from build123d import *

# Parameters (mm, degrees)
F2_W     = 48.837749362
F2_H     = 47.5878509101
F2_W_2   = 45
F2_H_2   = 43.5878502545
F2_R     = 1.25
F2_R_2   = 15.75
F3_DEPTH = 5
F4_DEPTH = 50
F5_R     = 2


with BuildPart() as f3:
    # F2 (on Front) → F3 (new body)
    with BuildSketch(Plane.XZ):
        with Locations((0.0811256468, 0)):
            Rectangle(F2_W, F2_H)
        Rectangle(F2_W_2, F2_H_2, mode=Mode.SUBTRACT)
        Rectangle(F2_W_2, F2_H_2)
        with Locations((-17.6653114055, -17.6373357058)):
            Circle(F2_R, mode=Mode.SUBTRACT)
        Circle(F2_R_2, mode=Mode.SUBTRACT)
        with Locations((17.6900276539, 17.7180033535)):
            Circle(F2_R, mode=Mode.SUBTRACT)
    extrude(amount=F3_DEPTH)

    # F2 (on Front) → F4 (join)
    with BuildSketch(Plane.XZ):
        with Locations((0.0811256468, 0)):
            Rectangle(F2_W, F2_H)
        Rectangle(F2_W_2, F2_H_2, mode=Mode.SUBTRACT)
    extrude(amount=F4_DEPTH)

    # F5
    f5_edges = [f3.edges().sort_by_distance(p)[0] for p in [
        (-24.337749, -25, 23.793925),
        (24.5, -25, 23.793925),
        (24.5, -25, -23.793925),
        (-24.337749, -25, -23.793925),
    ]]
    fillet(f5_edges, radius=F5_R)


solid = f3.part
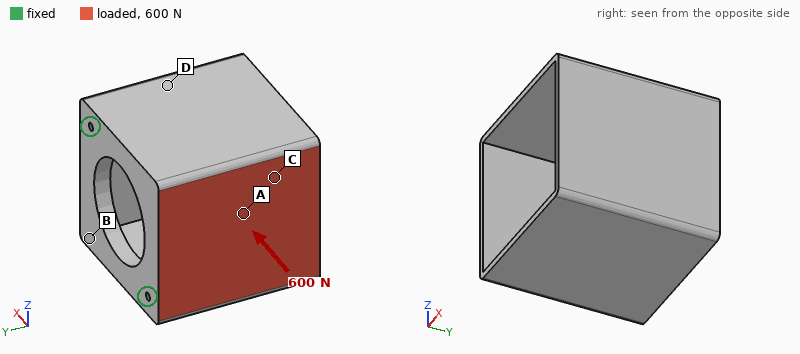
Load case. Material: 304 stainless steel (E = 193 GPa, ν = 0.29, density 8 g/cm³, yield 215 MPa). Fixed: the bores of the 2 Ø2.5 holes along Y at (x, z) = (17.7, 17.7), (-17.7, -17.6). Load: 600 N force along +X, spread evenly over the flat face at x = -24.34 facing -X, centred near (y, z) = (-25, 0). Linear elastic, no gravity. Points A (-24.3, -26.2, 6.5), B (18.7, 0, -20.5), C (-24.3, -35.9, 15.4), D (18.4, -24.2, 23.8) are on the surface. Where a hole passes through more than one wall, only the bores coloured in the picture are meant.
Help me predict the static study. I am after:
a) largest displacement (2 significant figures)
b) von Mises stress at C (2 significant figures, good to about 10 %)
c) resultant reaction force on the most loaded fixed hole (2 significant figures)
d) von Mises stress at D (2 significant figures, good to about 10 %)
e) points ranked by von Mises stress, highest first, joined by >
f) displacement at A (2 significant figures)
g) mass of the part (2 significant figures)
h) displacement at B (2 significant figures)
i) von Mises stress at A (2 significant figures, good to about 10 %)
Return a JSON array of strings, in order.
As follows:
["89 µm", "17 MPa", "350 N", "12 MPa", "A > C > D > B", "46 µm", "190 g", "16 µm", "33 MPa"]
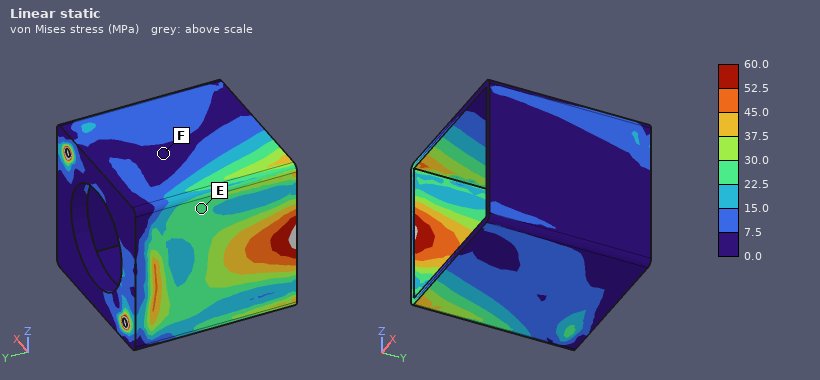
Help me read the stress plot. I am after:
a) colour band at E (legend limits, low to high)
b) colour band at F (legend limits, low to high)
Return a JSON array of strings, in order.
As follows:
["22.5 to 30.0 MPa", "0.0 to 7.5 MPa"]
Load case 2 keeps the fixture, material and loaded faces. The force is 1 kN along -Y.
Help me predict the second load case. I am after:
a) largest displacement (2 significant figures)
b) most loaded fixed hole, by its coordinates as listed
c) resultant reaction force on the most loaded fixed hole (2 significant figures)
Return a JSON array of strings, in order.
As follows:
["97 µm", "(-17.7, -17.6)", "810 N"]
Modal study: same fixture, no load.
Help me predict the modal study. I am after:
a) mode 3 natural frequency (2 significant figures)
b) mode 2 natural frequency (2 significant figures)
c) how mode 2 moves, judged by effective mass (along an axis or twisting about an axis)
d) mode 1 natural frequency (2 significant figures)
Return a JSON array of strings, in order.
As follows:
["2700 Hz", "1900 Hz", "along Y", "1500 Hz"]
